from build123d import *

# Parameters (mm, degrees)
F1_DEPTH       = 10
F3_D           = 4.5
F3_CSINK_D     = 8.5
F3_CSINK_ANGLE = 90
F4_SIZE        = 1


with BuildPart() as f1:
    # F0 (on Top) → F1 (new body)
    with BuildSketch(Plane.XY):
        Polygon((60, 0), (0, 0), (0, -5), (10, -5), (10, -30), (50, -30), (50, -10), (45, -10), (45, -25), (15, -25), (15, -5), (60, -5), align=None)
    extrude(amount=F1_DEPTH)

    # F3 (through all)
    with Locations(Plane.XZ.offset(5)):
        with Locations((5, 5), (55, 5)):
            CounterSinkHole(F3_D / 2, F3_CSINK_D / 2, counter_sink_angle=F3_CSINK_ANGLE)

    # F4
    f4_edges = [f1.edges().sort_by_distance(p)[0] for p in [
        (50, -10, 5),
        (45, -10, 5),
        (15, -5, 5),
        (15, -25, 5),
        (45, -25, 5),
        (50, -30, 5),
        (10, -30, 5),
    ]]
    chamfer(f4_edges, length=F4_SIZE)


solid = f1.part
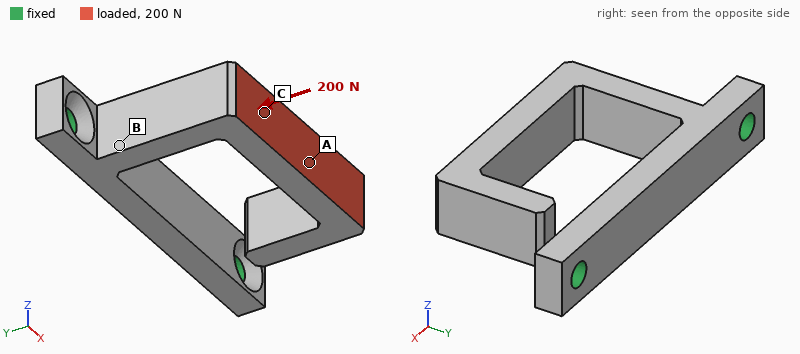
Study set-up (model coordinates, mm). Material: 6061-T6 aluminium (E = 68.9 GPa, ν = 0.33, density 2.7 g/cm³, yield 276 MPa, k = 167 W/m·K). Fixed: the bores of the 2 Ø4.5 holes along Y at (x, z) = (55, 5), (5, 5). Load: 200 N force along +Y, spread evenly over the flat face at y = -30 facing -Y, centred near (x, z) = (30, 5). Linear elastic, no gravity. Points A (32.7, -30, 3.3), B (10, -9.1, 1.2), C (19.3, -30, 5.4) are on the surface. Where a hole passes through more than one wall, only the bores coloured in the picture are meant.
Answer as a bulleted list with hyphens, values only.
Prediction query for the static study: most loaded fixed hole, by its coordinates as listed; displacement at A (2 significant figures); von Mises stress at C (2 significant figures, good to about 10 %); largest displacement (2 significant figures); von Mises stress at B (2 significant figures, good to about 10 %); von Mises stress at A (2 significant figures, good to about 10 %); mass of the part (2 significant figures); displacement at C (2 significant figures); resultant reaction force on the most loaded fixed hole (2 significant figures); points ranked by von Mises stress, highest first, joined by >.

- (5, 5)
- 0.41 mm
- 55 MPa
- 0.69 mm
- 79 MPa
- 17 MPa
- 18 g
- 0.26 mm
- 180 N
- B > C > A
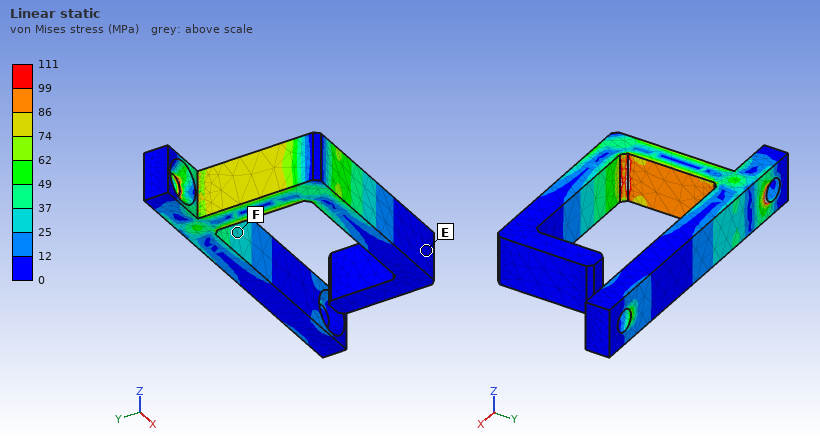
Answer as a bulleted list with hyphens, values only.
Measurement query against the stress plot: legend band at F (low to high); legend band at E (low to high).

- 25 to 37 MPa
- 0 to 12 MPa
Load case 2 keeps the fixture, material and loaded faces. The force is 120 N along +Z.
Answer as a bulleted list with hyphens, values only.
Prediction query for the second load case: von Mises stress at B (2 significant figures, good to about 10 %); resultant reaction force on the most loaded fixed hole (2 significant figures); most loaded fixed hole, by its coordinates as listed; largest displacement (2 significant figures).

- 43 MPa
- 84 N
- (5, 5)
- 0.33 mm
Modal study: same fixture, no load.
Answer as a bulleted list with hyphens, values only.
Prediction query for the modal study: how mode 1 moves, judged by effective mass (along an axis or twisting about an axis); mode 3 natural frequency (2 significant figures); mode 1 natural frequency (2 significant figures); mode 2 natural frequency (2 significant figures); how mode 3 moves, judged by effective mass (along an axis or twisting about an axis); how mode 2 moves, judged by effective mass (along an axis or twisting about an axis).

- along Y
- 2700 Hz
- 950 Hz
- 1200 Hz
- along X
- along Z
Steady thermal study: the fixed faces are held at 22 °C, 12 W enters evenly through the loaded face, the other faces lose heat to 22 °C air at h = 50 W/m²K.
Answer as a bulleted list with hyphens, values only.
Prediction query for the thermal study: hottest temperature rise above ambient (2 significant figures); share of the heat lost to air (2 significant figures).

- 46 K
- 28 %
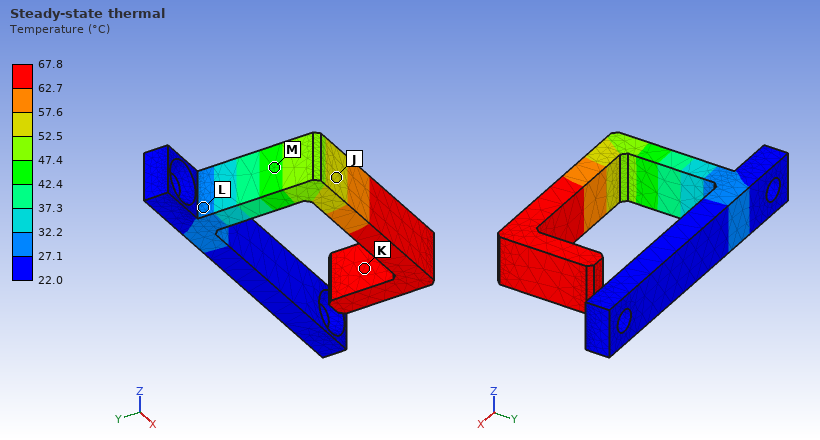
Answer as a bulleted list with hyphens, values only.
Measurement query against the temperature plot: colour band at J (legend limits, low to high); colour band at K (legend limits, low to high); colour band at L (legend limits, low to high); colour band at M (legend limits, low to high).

- 52.5 to 57.6 °C
- 62.7 to 67.8 °C
- 27.1 to 32.2 °C
- 42.4 to 47.4 °C
